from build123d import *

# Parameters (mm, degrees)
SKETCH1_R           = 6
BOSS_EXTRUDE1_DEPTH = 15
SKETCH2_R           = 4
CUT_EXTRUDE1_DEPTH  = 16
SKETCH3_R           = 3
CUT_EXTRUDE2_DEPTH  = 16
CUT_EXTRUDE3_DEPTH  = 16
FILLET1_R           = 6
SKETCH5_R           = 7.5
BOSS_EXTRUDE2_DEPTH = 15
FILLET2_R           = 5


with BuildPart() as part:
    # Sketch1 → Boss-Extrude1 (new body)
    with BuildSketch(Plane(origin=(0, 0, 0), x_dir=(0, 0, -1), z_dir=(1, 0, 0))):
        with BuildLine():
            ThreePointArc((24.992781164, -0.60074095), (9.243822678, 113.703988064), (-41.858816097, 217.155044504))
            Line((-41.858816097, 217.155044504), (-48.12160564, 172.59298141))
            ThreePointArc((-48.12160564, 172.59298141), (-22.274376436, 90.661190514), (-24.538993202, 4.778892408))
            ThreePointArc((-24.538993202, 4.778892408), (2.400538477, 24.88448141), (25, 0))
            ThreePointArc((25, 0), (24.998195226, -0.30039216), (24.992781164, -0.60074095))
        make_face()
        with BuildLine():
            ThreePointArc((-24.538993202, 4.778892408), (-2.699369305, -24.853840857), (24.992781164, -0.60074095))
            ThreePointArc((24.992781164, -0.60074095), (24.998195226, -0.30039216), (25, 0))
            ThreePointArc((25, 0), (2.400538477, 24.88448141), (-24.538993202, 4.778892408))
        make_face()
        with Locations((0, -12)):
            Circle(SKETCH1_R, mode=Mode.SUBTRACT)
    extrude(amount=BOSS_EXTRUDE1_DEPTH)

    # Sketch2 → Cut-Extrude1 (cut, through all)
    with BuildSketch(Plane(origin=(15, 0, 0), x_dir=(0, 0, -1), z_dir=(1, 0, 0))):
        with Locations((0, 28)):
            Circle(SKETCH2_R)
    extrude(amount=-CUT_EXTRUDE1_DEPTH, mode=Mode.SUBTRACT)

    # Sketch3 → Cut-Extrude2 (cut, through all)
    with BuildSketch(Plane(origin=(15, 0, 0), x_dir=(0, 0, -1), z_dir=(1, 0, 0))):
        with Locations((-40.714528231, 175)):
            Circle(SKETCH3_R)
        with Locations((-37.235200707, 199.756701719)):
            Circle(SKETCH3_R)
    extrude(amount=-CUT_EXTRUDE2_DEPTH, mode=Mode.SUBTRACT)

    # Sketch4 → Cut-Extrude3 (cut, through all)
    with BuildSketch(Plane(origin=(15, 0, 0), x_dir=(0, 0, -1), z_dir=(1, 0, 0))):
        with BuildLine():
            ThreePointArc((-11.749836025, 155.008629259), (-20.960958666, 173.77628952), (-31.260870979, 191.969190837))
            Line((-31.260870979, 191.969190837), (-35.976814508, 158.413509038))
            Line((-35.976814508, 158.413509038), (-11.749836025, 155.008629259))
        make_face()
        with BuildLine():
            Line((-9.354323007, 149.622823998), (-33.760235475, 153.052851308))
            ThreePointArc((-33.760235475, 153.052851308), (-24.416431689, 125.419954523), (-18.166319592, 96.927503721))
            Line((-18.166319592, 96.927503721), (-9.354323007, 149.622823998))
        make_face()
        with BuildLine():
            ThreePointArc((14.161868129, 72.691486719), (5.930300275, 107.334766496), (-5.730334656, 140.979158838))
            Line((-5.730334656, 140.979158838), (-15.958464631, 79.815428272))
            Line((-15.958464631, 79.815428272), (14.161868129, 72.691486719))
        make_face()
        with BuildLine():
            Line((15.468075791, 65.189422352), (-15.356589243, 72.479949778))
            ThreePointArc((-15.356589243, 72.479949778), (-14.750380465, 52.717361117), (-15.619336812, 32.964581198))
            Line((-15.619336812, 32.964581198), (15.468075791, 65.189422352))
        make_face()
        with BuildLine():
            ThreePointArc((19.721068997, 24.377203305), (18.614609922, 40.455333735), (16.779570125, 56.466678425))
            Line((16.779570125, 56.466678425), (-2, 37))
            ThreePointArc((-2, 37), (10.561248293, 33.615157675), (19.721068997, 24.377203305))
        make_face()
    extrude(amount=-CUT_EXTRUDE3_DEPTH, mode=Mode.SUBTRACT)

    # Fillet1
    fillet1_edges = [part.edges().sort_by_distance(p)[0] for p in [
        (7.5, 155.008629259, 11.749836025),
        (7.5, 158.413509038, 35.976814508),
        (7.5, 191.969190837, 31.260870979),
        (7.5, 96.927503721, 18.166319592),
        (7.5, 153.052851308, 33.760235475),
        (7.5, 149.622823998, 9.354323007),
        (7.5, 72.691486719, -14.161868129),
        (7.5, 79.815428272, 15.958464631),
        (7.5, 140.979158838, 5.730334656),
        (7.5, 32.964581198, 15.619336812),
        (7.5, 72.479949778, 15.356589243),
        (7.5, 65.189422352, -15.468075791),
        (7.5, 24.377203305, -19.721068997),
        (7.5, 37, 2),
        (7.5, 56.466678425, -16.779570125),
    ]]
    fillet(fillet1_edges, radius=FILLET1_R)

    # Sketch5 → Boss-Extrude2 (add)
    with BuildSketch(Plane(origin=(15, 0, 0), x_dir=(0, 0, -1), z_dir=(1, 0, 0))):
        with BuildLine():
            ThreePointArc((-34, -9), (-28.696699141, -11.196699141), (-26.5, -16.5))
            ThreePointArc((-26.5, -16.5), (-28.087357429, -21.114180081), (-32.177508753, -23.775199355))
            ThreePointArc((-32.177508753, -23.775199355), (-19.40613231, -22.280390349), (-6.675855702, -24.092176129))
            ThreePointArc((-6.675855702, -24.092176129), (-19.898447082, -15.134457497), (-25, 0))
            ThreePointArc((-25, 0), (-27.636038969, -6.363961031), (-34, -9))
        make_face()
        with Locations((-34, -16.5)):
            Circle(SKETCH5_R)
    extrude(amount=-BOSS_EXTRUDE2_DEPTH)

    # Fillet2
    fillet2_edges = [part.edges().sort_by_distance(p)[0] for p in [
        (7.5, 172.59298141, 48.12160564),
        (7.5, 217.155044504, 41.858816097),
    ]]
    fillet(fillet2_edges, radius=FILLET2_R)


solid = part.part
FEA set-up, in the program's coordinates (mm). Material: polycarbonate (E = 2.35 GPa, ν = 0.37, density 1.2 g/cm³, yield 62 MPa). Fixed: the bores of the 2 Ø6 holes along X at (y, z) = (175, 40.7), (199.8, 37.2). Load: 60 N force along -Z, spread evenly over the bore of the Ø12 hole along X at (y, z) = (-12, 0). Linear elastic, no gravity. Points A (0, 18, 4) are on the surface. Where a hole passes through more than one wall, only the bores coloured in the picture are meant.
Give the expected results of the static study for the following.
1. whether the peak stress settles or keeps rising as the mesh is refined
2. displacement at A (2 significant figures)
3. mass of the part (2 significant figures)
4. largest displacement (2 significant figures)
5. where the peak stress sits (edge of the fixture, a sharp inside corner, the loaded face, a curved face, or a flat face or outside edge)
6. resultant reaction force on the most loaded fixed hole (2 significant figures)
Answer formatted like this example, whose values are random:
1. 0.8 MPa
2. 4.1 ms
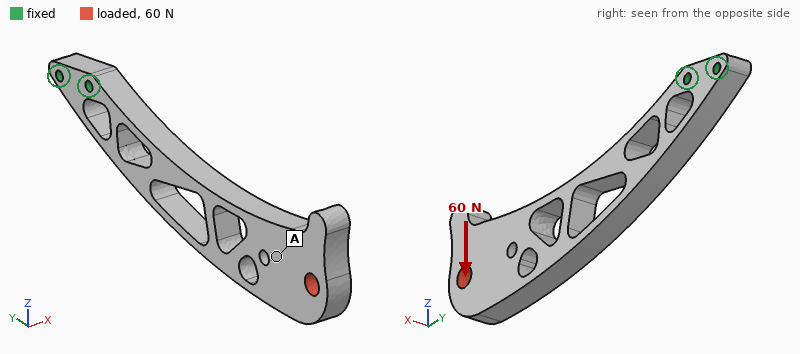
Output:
1. keeps rising
2. 2.2 mm
3. 110 g
4. 2.9 mm
5. edge of the fixture
6. 470 N
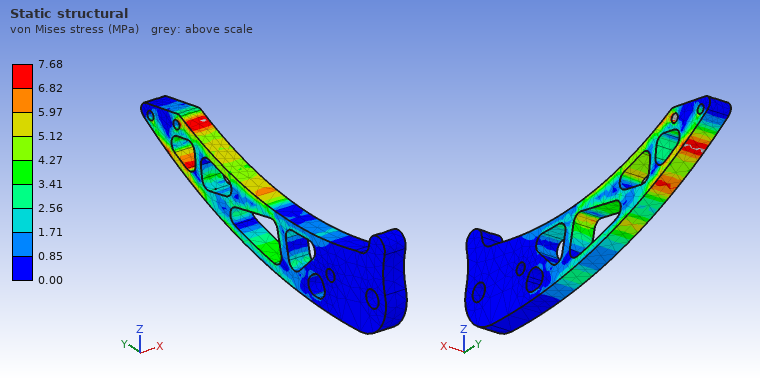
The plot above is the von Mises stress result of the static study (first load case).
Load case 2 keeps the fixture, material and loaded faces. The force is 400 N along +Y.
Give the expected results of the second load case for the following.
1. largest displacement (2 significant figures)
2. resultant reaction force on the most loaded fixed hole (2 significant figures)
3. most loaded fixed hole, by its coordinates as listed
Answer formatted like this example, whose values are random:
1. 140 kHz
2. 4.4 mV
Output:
1. 2.7 mm
2. 630 N
3. (199.8, 37.2)
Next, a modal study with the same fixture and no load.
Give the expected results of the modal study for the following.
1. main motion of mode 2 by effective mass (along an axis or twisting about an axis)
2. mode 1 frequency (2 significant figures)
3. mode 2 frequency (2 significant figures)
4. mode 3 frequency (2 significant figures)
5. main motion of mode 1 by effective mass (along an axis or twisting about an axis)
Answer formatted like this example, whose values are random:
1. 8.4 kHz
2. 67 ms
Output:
1. along Z
2. 47 Hz
3. 110 Hz
4. 220 Hz
5. along X
